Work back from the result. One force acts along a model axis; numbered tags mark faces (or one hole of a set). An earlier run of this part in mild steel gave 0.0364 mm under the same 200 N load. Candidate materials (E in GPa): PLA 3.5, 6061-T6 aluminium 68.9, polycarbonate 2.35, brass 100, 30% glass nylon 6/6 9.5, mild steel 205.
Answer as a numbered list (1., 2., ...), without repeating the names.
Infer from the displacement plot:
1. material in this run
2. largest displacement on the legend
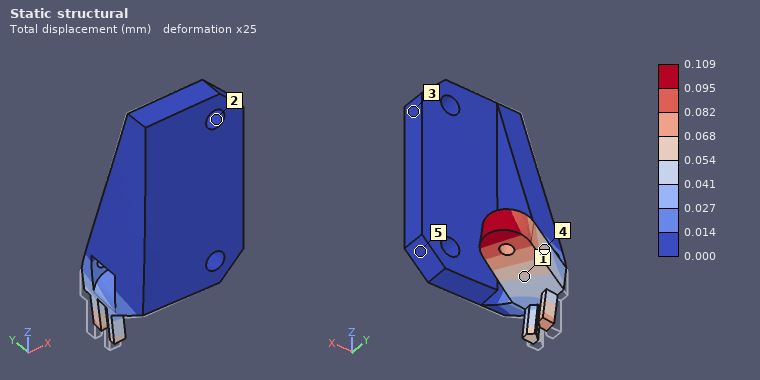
1. 6061-T6 aluminium
2. 0.109 mm
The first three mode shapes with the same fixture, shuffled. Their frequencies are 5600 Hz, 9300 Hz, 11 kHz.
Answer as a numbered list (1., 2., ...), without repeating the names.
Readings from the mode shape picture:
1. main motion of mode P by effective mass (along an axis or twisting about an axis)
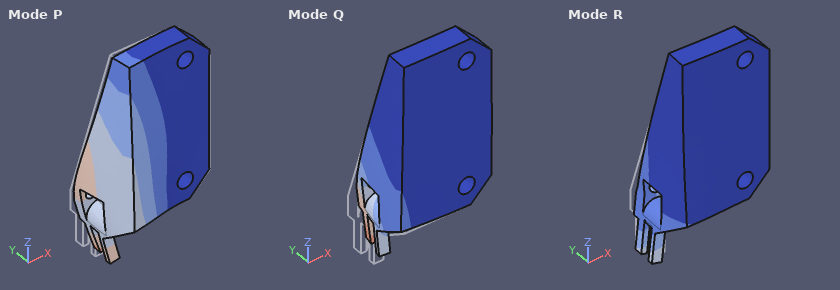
1. along Y
